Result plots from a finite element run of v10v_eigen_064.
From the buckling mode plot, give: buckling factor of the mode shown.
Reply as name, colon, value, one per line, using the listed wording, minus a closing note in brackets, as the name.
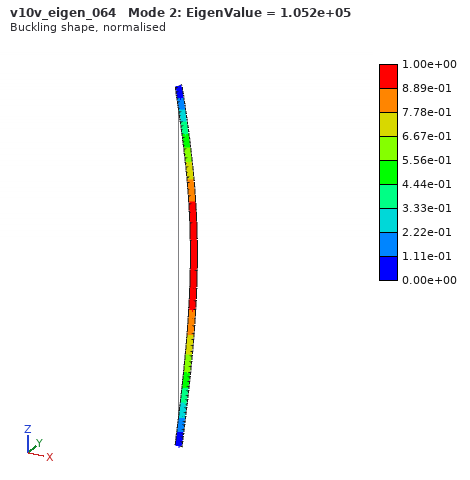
buckling factor of the mode shown: 1.052e+05
